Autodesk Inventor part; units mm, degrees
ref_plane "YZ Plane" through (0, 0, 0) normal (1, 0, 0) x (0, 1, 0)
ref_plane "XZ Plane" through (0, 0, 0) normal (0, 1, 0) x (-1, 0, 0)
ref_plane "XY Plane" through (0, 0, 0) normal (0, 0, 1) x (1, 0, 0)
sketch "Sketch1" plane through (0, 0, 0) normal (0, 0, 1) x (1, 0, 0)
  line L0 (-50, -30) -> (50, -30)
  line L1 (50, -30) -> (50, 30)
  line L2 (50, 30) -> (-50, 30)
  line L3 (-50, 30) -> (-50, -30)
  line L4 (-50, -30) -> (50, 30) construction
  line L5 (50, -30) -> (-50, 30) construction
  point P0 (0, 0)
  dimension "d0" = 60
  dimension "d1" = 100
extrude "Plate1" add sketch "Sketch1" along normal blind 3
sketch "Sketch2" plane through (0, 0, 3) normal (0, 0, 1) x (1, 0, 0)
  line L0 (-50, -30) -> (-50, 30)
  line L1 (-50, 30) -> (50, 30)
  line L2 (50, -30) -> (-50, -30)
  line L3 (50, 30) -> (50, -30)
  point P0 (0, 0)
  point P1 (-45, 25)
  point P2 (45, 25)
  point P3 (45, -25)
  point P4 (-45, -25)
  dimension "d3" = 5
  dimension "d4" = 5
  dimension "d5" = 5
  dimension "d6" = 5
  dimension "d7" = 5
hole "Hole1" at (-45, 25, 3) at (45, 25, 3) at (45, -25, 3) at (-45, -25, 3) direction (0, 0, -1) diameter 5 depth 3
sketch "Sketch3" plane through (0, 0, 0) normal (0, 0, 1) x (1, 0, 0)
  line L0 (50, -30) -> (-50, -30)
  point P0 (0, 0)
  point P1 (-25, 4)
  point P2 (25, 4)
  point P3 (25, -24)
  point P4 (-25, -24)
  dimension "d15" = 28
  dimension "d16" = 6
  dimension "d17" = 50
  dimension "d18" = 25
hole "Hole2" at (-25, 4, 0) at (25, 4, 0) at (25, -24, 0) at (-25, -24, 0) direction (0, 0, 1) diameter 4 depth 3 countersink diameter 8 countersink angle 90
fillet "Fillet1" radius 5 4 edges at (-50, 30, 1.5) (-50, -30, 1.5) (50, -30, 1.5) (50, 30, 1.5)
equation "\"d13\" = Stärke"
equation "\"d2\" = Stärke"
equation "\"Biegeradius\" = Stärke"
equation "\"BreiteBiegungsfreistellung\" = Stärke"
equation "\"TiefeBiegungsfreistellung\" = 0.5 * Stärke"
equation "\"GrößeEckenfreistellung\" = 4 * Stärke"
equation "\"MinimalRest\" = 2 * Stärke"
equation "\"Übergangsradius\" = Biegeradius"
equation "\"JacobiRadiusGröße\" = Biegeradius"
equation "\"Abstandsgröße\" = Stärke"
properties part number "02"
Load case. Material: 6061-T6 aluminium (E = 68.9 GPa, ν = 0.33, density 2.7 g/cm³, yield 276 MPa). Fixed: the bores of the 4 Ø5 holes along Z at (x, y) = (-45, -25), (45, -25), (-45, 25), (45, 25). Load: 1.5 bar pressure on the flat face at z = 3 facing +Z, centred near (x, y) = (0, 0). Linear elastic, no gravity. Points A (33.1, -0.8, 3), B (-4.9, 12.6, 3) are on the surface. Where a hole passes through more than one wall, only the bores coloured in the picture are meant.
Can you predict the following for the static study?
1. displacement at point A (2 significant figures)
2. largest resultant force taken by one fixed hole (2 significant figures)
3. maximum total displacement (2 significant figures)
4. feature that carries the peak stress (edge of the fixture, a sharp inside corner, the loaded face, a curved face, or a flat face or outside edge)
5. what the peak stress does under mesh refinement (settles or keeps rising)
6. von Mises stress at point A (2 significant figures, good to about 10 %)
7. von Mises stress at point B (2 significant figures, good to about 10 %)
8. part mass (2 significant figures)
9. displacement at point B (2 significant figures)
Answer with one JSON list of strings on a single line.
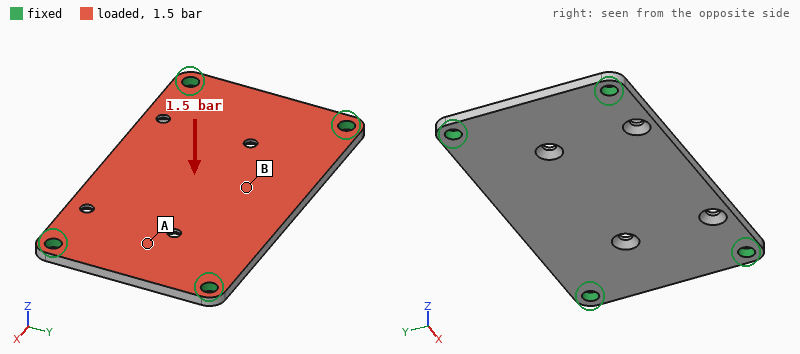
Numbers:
["0.077 mm", "220 N", "0.20 mm", "edge of the fixture", "keeps rising", "17 MPa", "32 MPa", "47 g", "0.20 mm"]
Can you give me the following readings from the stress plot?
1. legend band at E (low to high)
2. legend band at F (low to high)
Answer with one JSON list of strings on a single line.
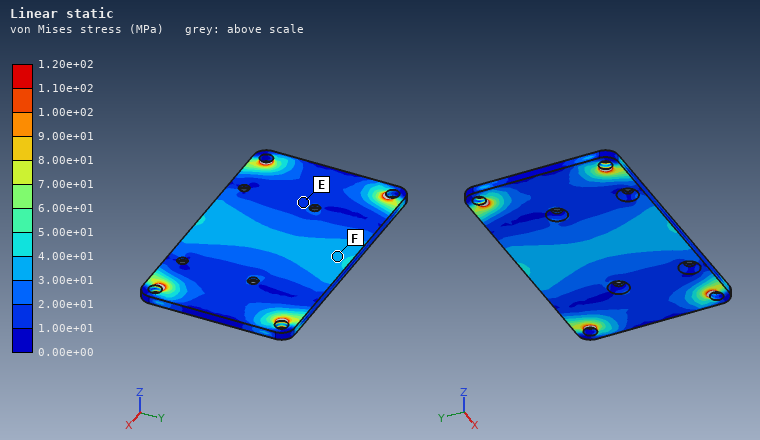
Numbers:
["1.00e+01 to 2.00e+01 MPa", "3.00e+01 to 4.00e+01 MPa"]
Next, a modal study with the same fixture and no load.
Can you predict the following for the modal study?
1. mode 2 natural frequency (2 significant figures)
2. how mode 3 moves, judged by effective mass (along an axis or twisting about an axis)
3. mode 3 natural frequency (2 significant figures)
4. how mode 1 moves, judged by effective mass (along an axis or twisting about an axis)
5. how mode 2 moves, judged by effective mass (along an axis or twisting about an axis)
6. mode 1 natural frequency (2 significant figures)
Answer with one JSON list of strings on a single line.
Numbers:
["2800 Hz", "twisting about Y", "4600 Hz", "along Z", "twisting about X", "1700 Hz"]
